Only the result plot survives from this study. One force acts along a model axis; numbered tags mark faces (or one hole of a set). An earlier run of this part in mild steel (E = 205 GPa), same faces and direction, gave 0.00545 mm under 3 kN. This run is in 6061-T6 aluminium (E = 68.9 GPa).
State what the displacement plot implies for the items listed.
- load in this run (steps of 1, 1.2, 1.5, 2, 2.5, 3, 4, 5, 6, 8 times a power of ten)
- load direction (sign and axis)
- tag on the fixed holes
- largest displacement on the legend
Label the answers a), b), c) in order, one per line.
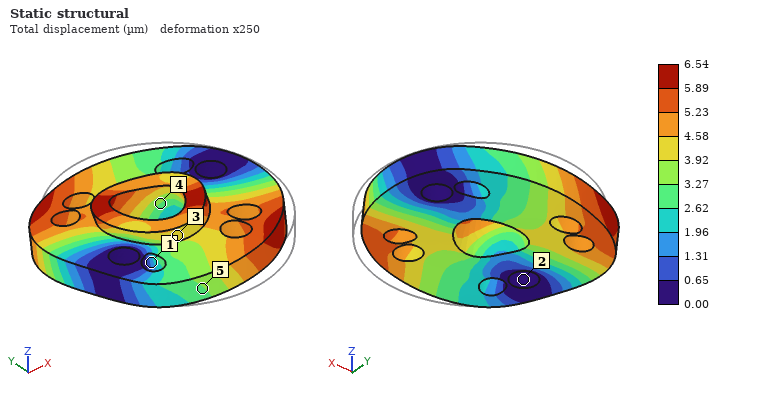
a) 1.2 kN
b) -X
c) 2
d) 6.54 µm
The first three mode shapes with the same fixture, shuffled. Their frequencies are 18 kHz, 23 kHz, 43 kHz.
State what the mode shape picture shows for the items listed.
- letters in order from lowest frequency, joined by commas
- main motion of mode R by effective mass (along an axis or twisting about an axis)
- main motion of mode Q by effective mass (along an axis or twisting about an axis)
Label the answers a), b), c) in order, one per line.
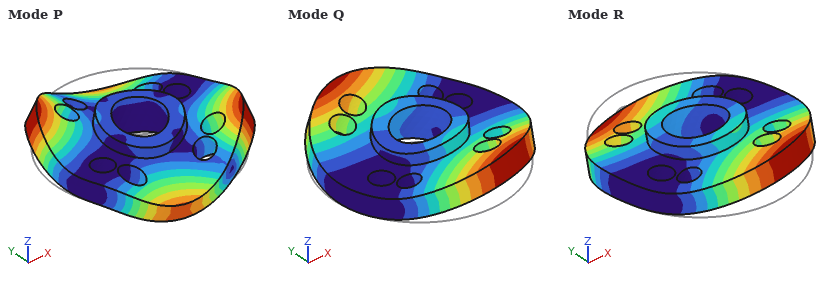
a) R, Q, P
b) twisting about X
c) along Z
